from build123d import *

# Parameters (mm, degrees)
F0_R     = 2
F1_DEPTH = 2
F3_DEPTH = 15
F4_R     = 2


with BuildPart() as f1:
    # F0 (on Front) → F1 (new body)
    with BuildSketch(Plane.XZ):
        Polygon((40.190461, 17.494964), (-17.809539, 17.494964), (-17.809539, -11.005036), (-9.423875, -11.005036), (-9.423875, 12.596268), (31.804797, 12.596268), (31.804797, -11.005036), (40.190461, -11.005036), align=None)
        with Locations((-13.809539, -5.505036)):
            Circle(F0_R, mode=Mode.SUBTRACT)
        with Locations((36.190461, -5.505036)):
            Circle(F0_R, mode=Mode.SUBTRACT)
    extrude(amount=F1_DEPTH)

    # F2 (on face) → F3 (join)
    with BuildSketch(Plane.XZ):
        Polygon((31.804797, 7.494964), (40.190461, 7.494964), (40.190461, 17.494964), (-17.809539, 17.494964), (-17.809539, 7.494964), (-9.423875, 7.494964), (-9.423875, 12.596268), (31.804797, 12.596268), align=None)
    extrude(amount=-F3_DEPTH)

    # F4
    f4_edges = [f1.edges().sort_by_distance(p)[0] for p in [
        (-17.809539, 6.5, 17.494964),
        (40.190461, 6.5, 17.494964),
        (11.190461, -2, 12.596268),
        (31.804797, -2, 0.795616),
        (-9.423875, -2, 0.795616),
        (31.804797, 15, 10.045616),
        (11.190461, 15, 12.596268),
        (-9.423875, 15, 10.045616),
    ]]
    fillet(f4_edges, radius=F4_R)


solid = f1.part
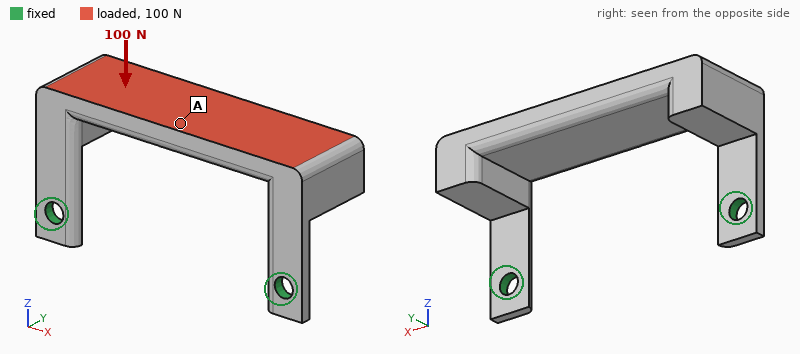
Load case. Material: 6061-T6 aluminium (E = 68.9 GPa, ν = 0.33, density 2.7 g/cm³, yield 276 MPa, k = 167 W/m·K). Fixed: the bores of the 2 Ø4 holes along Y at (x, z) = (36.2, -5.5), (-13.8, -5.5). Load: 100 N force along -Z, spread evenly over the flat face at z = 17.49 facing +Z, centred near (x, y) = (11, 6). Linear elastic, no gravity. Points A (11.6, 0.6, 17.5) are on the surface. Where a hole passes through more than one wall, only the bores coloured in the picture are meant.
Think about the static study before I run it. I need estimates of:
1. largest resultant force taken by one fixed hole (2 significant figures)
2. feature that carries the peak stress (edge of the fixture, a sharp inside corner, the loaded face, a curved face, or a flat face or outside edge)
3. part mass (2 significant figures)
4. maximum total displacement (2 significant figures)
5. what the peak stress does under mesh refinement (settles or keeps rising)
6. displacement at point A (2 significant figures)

52 N
edge of the fixture
18 g
0.28 mm
keeps rising
0.20 mm
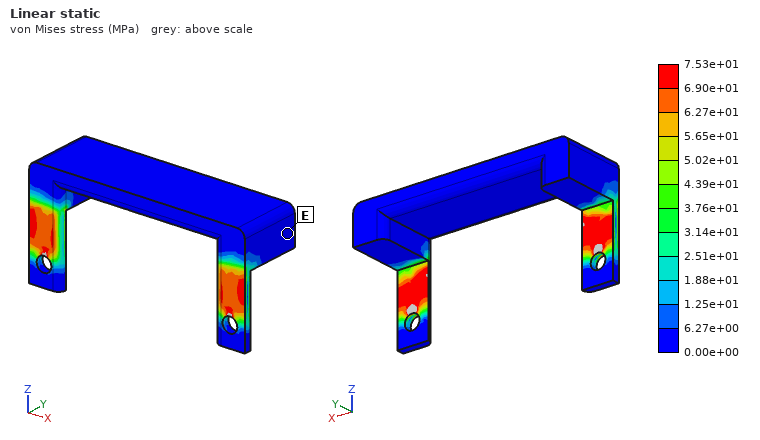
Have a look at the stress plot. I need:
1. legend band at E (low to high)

0.00e+00 to 6.27e+00 MPa
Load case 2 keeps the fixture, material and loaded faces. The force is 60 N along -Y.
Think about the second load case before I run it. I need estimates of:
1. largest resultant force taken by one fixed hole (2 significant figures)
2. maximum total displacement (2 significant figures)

31 N
0.36 mm
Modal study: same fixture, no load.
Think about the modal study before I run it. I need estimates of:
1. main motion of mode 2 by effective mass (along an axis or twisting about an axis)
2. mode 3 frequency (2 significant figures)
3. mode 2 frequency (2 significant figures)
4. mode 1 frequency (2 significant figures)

along X
3900 Hz
2600 Hz
620 Hz
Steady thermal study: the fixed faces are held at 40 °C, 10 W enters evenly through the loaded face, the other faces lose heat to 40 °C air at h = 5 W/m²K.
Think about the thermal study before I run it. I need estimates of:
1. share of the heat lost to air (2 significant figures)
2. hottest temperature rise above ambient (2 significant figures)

3.2 %
30 K
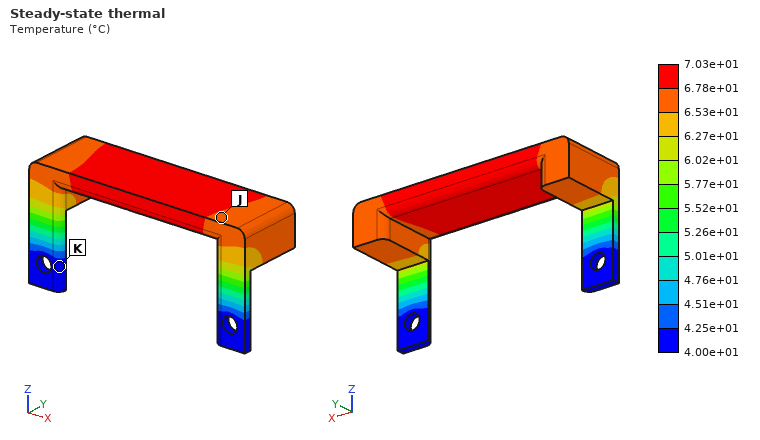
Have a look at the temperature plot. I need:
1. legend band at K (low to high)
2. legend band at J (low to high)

4.00e+01 to 4.25e+01 °C
6.53e+01 to 6.78e+01 °C
